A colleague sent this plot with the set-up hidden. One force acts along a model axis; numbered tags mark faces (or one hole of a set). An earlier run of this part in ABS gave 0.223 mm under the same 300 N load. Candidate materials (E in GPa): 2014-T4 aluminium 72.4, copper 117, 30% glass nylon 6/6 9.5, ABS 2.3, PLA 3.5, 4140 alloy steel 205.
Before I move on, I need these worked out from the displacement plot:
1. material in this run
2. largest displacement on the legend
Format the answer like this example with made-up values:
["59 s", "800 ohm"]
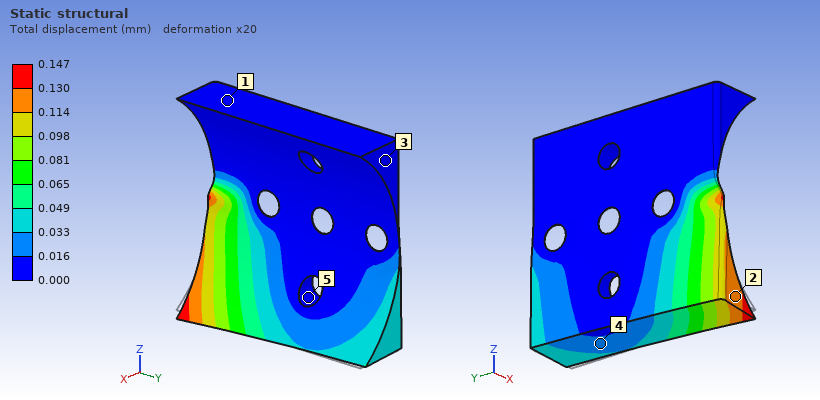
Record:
["PLA", "0.147 mm"]
